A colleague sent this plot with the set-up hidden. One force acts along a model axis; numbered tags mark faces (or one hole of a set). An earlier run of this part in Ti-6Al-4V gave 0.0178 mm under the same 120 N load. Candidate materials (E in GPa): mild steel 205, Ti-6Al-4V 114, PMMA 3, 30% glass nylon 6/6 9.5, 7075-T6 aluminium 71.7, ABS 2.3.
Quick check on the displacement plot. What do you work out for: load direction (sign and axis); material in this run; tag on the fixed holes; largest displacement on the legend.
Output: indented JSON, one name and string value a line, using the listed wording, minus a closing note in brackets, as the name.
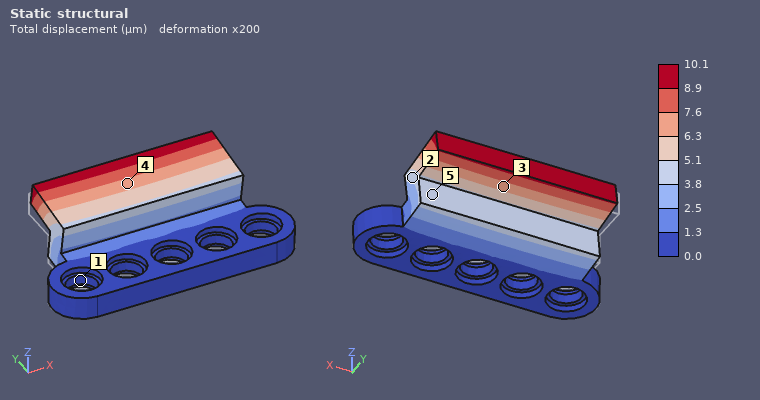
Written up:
{
  "load direction": "+Z",
  "material in this run": "mild steel",
  "tag on the fixed holes": "1",
  "largest displacement on the legend": "10.1 µm"
}
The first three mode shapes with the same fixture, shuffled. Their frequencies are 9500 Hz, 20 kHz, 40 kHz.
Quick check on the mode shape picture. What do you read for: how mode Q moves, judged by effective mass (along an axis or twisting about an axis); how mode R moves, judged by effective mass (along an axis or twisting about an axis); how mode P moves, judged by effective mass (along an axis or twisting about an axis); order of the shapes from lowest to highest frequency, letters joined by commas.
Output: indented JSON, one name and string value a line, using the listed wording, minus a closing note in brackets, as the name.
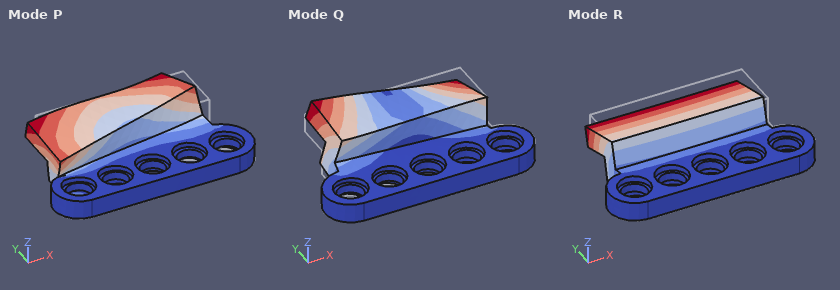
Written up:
{
  "how mode Q moves, judged by effective mass": "twisting about Y",
  "how mode R moves, judged by effective mass": "along Z",
  "how mode P moves, judged by effective mass": "along X",
  "order of the shapes from lowest to highest frequency, letters joined by commas": "R, Q, P"
}
